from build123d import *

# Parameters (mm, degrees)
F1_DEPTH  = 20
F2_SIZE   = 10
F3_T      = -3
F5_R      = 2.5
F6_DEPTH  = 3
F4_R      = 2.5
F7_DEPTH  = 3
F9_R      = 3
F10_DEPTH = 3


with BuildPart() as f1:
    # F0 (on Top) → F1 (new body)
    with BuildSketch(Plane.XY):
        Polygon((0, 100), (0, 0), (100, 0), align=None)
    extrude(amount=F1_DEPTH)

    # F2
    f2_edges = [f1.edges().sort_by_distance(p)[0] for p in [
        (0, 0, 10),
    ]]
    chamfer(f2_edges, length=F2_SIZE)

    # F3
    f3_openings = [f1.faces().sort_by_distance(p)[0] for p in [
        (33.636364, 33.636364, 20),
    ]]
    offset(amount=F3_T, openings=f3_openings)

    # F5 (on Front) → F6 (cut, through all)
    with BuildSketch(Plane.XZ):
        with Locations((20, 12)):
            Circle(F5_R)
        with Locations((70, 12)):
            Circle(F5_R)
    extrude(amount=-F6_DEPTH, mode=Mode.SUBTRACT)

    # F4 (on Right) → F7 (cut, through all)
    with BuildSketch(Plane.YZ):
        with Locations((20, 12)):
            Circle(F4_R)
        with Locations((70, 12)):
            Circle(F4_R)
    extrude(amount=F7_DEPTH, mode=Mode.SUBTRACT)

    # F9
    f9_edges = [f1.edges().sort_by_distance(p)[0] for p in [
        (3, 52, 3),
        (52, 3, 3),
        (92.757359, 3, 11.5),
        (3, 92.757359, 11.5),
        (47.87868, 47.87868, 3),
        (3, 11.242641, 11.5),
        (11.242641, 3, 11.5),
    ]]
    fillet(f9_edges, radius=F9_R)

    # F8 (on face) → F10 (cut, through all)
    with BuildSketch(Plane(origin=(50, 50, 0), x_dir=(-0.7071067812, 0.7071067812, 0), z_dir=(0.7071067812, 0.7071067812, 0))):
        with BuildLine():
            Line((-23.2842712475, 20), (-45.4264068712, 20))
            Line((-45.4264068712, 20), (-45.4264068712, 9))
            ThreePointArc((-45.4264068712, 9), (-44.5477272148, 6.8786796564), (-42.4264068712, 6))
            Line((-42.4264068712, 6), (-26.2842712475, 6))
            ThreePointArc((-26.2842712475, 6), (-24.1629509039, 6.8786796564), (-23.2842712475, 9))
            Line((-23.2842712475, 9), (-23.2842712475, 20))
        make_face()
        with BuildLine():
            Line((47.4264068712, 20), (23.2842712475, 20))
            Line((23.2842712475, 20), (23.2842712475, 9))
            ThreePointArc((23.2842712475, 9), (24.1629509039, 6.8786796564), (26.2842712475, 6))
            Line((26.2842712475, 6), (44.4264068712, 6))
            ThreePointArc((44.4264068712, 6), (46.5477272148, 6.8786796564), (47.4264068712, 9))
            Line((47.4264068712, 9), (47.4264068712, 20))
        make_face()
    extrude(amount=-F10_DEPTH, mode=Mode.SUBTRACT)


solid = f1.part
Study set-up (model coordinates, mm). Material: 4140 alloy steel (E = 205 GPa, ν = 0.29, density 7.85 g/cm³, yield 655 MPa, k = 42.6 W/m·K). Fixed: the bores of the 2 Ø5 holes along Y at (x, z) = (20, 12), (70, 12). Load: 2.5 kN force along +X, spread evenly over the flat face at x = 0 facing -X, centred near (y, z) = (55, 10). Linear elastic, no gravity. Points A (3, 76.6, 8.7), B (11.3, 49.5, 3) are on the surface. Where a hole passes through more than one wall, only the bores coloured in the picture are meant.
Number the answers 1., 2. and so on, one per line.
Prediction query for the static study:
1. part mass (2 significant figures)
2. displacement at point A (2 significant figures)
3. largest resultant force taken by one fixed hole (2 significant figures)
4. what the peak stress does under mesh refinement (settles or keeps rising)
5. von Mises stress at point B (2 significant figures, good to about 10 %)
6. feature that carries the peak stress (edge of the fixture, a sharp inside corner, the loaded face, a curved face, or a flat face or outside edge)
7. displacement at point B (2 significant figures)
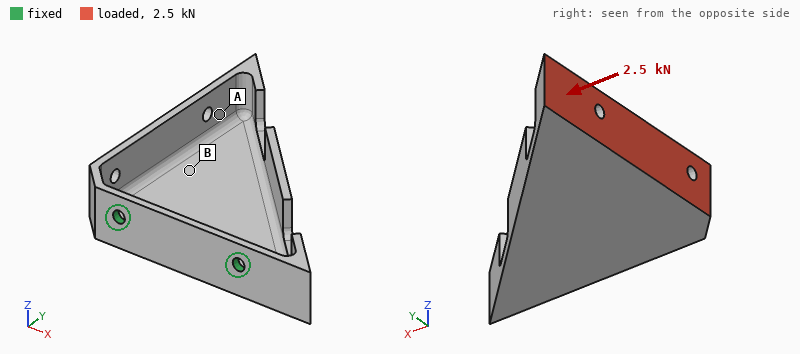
1. 230 g
2. 0.36 mm
3. 2.9 kN
4. keeps rising
5. 110 MPa
6. edge of the fixture
7. 0.16 mm
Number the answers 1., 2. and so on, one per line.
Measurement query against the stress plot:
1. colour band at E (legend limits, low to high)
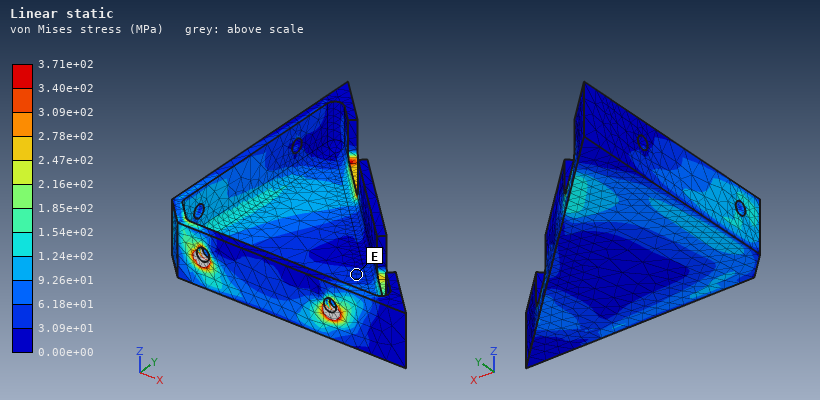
1. 3.09e+01 to 6.18e+01 MPa
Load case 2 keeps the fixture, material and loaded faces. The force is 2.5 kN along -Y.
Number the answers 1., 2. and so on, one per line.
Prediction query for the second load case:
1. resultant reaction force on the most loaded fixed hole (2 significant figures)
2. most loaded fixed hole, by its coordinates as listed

1. 3.3 kN
2. (20, 12)
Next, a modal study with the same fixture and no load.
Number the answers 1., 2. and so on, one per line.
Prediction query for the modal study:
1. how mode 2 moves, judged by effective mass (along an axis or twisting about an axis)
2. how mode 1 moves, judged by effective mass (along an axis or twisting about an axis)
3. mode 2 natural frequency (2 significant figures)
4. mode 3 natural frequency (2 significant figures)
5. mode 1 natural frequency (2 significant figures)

1. along X
2. along Z
3. 1400 Hz
4. 2400 Hz
5. 420 Hz
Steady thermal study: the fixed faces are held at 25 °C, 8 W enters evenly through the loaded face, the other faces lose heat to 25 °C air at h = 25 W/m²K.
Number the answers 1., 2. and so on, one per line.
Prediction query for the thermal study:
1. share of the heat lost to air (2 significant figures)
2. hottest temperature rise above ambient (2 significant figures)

1. 63 %
2. 31 K
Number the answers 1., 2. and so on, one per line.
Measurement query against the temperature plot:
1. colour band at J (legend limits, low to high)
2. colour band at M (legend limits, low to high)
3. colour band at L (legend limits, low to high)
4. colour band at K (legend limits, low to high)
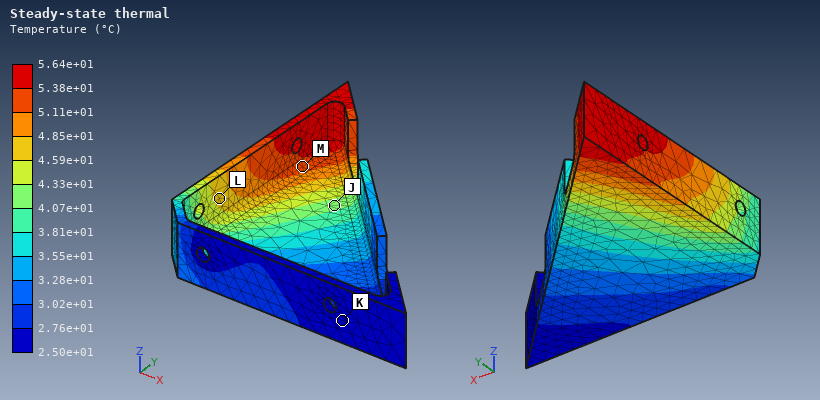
1. 4.07e+01 to 4.33e+01 °C
2. 5.11e+01 to 5.38e+01 °C
3. 4.59e+01 to 4.85e+01 °C
4. 2.50e+01 to 2.76e+01 °C
